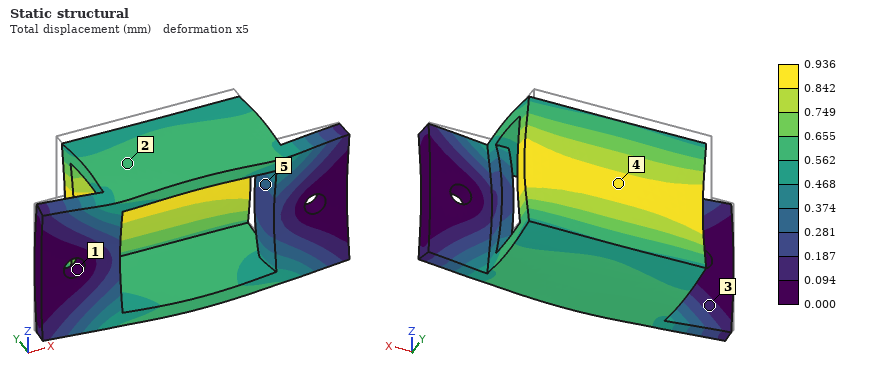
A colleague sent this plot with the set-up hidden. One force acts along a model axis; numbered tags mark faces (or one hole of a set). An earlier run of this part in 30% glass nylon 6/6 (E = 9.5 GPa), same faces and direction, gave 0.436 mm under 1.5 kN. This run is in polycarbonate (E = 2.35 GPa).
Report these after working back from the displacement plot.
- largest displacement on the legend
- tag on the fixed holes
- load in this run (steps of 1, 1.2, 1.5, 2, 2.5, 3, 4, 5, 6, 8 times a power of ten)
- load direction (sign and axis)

0.936 mm
1
800 N
-Y
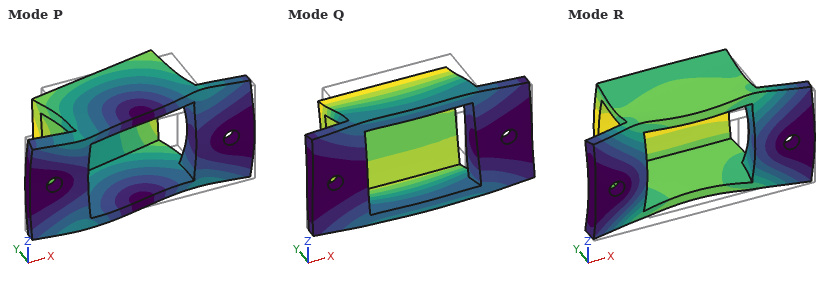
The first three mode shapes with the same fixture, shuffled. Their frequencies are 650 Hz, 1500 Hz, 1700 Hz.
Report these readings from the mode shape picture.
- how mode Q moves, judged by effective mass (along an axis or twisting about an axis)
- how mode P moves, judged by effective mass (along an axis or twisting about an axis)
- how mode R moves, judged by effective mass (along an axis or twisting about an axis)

along Z
along X
along Y
